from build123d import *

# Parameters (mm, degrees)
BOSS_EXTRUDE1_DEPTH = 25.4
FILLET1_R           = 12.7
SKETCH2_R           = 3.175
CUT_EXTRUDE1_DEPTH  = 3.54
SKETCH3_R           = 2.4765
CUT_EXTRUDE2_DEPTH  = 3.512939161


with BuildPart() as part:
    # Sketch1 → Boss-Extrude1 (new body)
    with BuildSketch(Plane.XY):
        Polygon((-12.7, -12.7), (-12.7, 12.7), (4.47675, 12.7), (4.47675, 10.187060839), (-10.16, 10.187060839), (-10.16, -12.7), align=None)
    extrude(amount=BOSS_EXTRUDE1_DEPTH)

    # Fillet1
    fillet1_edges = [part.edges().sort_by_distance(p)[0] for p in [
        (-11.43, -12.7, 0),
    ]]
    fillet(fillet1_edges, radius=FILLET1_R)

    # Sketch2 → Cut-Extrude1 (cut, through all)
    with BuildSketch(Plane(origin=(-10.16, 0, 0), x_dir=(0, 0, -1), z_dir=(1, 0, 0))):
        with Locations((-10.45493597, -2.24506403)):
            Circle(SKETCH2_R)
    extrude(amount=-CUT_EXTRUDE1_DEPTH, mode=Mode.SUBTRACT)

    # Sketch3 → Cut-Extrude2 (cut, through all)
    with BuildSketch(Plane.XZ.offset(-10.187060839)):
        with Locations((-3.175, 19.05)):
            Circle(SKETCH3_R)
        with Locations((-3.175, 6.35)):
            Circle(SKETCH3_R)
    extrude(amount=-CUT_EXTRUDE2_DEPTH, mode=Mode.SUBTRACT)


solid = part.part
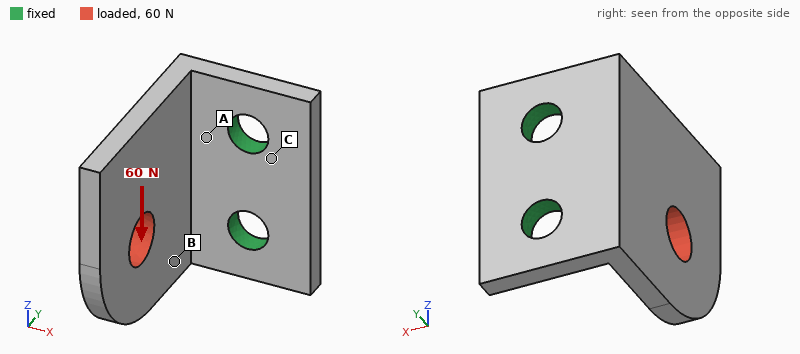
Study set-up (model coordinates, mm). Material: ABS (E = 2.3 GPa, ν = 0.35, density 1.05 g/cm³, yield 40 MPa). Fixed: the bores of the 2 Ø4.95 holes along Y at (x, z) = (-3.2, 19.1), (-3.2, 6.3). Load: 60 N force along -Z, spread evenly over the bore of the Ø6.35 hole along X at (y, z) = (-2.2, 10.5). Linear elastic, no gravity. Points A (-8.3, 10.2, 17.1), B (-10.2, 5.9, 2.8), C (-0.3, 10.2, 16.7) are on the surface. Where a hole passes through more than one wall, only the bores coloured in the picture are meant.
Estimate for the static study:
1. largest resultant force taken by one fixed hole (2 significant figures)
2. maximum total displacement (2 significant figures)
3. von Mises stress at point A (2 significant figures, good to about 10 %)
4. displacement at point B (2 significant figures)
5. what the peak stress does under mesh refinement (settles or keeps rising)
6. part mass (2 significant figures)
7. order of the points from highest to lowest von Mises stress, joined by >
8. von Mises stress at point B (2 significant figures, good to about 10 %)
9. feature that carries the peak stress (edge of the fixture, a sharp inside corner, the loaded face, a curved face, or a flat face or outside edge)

64 N
0.39 mm
9.0 MPa
0.15 mm
keeps rising
2.4 g
A > B > C
5.7 MPa
edge of the fixture
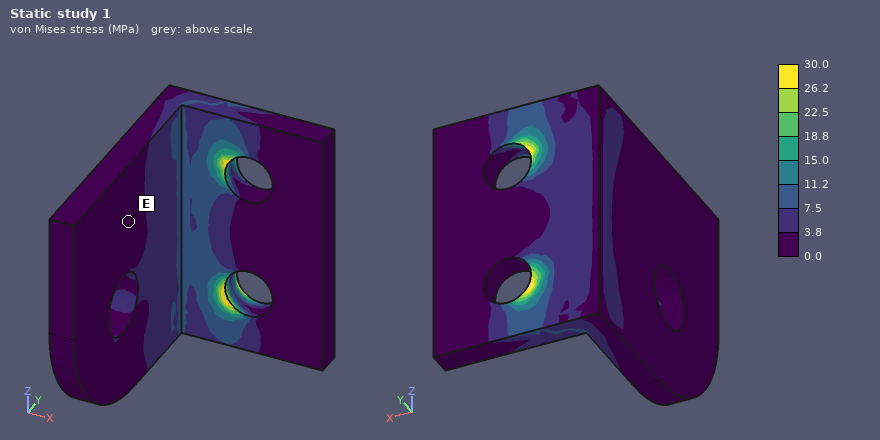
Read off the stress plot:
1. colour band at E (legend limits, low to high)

0.0 to 3.8 MPa
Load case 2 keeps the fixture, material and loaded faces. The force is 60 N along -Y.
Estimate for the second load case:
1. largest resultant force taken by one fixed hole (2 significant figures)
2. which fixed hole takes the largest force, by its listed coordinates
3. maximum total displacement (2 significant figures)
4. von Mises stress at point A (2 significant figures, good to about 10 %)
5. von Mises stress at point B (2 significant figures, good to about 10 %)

38 N
(-3.2, 6.3)
0.42 mm
6.3 MPa
1.8 MPa
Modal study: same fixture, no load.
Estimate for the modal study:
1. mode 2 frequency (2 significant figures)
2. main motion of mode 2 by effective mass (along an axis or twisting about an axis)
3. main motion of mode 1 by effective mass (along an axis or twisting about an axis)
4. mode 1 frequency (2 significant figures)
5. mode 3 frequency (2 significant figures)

2000 Hz
along Z
along X
830 Hz
2800 Hz
